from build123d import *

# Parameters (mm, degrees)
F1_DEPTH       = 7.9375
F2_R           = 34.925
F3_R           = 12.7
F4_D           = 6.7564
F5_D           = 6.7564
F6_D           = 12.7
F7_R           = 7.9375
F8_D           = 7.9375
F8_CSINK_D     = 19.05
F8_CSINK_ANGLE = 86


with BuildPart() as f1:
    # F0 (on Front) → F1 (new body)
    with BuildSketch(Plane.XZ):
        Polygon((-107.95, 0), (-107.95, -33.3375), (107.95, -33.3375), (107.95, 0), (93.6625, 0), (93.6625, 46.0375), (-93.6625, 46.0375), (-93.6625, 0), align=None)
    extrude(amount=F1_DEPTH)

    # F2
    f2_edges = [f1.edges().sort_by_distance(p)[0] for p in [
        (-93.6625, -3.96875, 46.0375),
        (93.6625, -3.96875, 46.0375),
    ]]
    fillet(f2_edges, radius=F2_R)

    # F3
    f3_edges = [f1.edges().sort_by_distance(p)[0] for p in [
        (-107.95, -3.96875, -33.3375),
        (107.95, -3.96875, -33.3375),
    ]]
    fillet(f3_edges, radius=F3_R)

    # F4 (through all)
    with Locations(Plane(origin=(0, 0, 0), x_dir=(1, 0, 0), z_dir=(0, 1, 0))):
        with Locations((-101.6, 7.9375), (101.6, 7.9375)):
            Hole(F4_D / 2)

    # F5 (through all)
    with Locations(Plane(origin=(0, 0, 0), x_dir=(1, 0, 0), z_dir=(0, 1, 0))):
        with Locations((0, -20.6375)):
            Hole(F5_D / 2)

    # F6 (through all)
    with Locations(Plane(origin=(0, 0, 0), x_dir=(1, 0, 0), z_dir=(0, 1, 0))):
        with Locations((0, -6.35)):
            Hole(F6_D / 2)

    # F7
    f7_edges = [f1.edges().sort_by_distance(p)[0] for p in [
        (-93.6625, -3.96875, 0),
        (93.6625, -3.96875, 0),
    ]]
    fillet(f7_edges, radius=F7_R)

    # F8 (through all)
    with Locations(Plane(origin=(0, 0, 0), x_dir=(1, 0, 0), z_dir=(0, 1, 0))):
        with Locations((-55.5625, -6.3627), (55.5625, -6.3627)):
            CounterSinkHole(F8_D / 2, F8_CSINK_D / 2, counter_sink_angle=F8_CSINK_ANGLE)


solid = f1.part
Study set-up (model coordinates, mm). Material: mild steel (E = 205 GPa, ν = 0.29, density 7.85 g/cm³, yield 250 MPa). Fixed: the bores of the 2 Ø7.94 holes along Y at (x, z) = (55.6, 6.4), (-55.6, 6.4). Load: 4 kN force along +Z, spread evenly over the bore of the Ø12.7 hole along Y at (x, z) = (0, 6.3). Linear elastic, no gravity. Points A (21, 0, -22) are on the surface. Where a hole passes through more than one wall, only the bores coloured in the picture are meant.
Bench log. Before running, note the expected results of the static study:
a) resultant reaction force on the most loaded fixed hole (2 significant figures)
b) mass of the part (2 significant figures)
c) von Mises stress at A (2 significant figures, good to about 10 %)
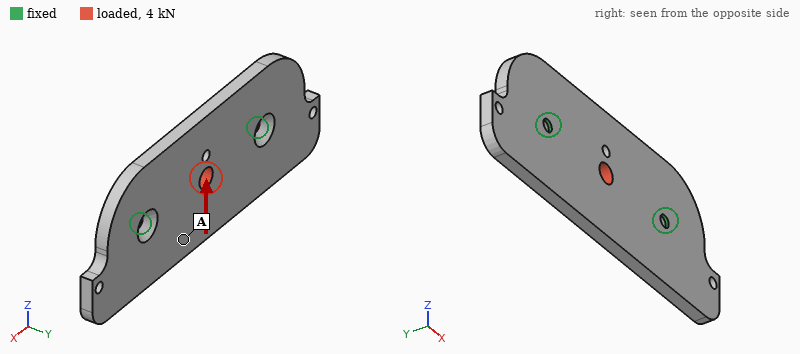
2.0 kN
920 g
7.3 MPa
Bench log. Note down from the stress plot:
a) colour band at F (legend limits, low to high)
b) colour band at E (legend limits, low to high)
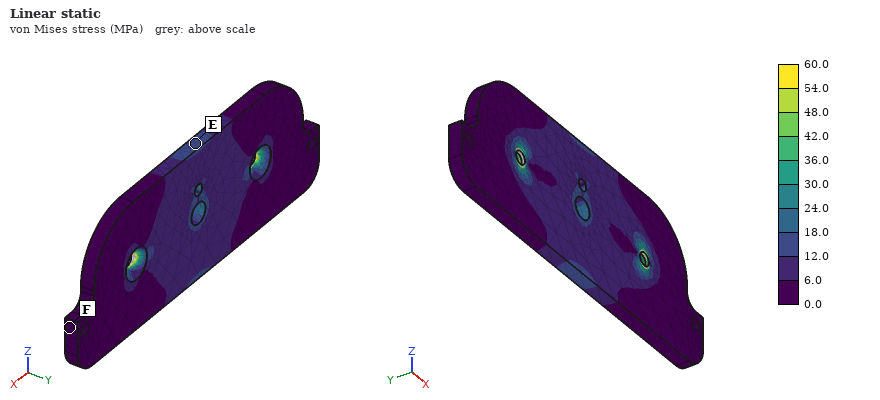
0.0 to 6.0 MPa
12.0 to 18.0 MPa
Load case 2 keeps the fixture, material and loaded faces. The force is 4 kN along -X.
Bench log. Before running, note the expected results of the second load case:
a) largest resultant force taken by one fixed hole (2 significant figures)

2.0 kN
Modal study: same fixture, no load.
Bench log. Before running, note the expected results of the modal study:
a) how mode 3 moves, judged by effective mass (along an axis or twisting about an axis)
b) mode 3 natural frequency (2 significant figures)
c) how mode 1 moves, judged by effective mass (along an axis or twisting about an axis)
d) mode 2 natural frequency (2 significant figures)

twisting about Z
1700 Hz
twisting about X
1600 Hz
